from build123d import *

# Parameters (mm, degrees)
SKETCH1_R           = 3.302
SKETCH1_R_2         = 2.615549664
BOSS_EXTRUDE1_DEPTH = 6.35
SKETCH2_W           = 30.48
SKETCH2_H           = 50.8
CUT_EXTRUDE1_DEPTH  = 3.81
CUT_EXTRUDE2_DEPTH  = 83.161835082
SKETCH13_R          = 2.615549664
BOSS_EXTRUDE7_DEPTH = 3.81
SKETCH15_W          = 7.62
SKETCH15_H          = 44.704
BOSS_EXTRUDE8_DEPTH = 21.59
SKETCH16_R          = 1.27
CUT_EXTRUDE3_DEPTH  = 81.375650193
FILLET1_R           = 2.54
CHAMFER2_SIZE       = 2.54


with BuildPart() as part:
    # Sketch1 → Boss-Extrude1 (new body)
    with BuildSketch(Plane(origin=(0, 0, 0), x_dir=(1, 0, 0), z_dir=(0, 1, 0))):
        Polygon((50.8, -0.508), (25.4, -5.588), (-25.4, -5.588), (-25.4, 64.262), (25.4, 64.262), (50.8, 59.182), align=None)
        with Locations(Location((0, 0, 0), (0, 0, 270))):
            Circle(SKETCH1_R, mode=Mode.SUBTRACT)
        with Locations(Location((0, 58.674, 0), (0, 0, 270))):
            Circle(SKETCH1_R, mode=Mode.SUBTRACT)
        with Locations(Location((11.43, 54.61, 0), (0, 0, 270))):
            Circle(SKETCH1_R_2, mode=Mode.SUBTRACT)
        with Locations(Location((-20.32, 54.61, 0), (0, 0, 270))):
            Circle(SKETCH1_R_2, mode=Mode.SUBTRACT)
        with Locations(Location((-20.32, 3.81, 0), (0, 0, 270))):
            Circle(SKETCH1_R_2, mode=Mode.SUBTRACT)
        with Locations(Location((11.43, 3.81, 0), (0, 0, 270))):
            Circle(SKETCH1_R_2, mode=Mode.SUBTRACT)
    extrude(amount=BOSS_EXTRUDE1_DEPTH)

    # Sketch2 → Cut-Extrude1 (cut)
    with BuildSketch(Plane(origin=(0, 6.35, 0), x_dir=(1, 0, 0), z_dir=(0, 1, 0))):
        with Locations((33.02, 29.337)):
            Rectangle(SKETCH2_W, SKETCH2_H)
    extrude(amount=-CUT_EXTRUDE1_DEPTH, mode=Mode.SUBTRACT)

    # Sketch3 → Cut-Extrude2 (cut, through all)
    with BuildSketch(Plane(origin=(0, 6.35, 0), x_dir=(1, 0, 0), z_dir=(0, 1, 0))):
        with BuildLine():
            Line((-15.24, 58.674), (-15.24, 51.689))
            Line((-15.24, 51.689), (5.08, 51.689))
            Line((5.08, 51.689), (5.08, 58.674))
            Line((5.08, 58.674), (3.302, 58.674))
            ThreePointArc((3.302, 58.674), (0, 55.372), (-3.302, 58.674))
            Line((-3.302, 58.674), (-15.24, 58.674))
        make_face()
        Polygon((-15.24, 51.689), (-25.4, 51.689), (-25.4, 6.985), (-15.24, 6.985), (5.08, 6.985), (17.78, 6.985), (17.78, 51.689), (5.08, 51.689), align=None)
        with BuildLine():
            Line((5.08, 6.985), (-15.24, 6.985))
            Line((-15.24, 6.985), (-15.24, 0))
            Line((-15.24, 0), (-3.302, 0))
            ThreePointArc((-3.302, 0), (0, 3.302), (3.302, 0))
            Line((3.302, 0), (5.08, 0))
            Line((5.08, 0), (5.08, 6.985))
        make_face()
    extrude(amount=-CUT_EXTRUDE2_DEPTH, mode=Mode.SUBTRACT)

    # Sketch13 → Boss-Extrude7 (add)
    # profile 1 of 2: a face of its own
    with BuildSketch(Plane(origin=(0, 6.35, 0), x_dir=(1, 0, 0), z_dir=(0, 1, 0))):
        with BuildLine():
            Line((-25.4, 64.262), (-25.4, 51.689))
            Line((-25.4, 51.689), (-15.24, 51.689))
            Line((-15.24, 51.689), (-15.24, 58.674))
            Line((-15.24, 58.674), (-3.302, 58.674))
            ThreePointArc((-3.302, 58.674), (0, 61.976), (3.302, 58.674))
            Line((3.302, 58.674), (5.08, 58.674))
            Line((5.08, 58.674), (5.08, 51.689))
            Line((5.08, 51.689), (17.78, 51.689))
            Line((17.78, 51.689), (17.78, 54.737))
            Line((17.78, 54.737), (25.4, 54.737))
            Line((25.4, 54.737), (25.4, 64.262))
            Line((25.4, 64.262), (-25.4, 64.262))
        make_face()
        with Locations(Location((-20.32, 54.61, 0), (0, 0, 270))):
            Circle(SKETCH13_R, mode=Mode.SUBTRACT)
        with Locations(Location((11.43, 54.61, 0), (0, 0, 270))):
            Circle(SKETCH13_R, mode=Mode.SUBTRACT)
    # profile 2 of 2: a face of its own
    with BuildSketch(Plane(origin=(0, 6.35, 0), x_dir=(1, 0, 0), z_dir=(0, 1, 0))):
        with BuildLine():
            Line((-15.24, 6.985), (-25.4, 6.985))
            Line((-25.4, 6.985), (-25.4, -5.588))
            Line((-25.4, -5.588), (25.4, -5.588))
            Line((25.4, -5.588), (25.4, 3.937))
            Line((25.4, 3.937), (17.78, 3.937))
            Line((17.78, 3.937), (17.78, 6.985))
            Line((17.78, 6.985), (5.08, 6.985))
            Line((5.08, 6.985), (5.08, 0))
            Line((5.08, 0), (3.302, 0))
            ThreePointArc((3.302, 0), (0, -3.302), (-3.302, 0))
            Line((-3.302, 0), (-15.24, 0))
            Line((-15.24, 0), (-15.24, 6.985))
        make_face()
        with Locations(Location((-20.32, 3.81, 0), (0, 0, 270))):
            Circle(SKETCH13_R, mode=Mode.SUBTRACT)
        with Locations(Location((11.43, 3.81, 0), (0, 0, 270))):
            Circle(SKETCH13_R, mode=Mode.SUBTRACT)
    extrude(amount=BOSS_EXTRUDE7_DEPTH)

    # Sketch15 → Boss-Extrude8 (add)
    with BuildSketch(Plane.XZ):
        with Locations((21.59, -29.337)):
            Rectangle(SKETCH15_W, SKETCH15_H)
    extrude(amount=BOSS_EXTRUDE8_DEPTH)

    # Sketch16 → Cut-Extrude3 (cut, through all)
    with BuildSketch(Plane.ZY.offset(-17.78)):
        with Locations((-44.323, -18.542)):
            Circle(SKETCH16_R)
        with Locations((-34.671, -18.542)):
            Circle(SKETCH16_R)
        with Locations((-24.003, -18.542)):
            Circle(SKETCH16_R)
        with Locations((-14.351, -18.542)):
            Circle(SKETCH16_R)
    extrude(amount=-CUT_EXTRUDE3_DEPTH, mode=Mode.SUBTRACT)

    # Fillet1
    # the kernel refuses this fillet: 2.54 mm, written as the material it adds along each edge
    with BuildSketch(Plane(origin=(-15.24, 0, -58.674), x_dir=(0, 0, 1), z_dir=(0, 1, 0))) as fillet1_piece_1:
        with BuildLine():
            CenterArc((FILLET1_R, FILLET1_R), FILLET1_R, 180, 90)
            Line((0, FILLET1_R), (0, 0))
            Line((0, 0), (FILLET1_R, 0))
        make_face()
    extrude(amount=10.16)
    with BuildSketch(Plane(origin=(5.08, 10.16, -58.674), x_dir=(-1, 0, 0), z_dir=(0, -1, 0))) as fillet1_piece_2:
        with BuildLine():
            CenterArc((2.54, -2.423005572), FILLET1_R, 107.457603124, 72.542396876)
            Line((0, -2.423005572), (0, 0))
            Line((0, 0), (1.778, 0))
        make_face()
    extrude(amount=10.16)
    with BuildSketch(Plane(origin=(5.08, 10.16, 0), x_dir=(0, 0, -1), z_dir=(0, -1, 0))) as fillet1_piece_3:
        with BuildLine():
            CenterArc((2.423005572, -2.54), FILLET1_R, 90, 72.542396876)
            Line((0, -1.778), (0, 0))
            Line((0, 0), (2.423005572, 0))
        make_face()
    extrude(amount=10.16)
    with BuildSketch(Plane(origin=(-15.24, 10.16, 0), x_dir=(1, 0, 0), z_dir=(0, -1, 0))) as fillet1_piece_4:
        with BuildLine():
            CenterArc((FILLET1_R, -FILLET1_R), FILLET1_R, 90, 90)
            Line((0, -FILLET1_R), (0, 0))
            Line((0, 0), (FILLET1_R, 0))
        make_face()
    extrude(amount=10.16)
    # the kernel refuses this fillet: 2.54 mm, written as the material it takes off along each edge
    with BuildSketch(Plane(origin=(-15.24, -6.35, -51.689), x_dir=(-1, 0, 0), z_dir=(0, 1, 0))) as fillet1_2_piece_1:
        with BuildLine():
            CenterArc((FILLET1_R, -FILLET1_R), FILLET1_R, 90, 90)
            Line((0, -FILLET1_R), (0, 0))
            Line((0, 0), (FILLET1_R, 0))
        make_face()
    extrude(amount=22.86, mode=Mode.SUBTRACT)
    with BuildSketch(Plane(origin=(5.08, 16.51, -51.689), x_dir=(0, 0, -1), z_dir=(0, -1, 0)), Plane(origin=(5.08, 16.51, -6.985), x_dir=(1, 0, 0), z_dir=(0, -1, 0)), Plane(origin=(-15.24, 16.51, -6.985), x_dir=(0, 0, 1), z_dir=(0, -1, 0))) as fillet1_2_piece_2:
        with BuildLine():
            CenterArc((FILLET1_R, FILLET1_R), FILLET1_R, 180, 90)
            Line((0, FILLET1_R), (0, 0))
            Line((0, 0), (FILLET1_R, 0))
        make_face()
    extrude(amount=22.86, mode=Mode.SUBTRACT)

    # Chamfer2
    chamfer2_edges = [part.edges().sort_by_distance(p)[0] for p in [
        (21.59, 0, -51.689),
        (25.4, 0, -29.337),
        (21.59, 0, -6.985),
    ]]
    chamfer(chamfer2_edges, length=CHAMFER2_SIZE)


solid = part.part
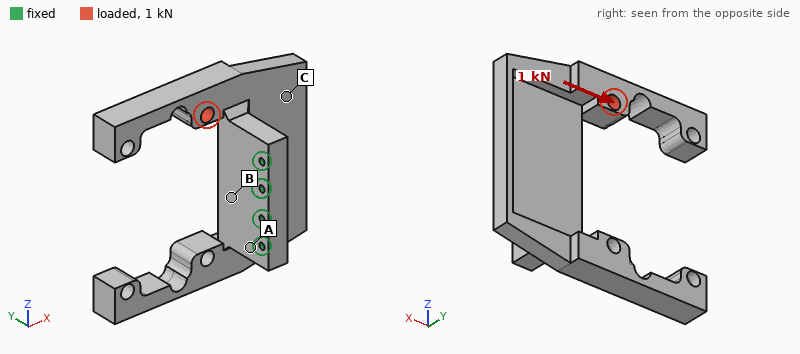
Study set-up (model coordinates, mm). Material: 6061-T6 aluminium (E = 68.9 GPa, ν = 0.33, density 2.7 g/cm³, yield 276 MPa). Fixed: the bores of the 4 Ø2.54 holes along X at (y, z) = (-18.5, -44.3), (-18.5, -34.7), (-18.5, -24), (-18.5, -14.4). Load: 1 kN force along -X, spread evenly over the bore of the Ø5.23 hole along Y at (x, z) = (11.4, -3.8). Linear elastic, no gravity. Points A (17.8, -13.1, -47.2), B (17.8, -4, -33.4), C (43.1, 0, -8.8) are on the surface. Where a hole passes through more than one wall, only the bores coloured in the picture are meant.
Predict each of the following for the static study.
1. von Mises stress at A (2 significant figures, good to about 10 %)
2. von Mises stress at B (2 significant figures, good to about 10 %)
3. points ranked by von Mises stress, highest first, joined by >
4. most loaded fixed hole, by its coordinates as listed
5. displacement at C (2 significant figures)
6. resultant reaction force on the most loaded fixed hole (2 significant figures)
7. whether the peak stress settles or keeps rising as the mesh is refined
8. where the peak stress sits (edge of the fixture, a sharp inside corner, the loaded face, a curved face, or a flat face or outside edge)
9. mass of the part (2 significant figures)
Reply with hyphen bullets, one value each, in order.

- 23 MPa
- 39 MPa
- B > A > C
- (-18.5, -14.4)
- 0.16 mm
- 850 N
- keeps rising
- edge of the fixture
- 62 g
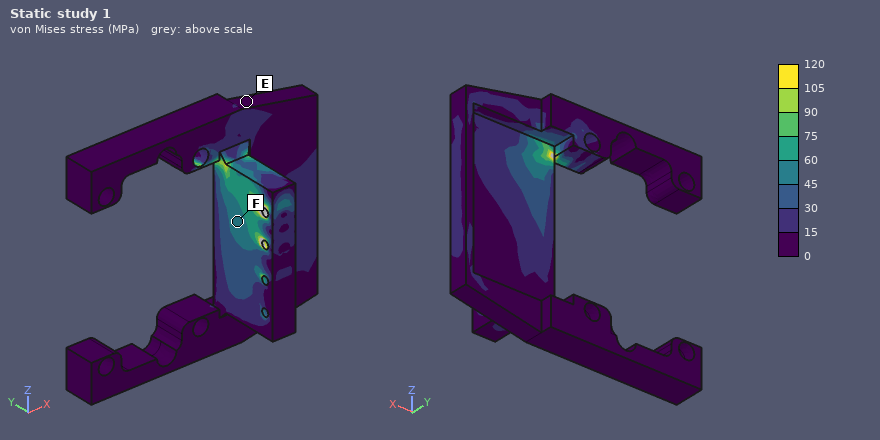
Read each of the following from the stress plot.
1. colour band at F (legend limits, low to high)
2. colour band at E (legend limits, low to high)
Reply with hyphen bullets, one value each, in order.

- 45 to 60 MPa
- 0 to 15 MPa
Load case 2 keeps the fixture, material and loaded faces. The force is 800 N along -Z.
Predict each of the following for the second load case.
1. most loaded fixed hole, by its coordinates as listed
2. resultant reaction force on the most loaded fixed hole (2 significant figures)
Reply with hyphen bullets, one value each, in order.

- (-18.5, -14.4)
- 750 N
